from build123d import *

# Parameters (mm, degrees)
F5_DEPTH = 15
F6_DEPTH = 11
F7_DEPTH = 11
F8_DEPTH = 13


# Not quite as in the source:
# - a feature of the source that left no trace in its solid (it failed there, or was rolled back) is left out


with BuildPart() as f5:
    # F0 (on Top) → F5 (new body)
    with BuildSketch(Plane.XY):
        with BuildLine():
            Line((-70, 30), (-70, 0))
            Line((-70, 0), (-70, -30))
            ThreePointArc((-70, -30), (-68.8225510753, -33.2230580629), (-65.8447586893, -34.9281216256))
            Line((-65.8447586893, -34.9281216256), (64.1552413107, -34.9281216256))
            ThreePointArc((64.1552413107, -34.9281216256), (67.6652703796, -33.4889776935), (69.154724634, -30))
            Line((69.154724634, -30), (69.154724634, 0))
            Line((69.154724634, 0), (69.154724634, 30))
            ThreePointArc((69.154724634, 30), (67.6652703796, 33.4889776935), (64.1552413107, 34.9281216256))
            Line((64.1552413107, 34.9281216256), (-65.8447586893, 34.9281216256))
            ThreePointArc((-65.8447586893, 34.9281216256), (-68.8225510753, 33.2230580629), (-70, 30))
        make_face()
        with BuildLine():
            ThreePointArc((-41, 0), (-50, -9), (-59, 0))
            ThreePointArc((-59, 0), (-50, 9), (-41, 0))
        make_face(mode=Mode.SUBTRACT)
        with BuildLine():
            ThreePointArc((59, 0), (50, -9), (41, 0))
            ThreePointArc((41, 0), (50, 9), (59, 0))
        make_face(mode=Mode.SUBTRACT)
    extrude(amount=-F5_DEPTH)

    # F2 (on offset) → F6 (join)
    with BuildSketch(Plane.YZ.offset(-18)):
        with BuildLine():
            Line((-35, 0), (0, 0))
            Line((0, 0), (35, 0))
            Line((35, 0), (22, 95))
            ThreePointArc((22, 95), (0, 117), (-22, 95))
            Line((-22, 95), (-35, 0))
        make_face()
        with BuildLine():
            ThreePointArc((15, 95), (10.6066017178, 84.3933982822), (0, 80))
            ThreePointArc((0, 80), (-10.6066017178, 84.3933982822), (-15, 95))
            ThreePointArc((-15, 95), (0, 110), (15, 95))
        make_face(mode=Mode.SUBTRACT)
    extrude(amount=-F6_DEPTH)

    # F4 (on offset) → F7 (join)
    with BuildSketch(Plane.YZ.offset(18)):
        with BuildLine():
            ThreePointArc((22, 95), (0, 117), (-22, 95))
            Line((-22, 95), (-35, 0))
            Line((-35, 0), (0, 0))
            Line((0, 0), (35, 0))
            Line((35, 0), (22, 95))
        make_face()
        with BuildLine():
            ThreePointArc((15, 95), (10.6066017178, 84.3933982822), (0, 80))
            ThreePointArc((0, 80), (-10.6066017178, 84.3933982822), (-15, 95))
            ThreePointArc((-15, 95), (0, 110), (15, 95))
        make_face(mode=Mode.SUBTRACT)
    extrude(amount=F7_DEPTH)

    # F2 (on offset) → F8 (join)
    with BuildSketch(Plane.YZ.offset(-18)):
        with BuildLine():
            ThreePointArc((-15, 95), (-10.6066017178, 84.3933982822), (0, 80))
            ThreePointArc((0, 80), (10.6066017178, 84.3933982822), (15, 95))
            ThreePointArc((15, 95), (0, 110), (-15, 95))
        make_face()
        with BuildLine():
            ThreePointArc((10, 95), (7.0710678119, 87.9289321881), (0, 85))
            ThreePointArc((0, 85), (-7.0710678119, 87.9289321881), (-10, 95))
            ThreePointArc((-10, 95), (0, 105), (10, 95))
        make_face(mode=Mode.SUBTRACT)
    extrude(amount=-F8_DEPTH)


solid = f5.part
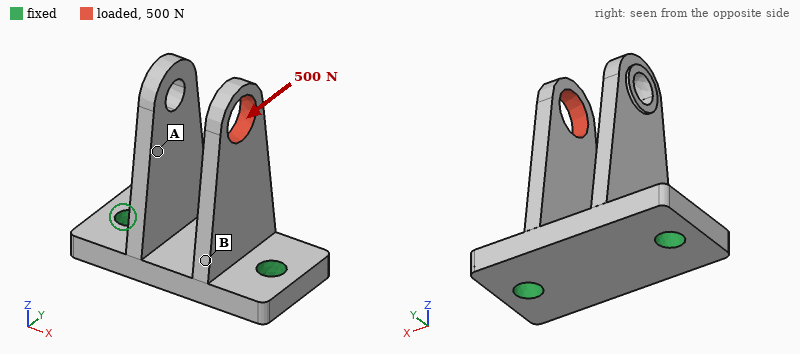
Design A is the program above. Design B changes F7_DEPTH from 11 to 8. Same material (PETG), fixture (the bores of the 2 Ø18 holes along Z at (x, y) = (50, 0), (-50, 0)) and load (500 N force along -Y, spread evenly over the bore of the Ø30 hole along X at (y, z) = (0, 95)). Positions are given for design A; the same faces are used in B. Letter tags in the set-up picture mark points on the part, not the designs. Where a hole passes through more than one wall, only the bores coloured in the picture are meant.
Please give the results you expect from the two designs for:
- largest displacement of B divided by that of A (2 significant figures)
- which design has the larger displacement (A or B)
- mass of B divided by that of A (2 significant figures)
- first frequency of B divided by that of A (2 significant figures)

1.2
B
0.94
0.88
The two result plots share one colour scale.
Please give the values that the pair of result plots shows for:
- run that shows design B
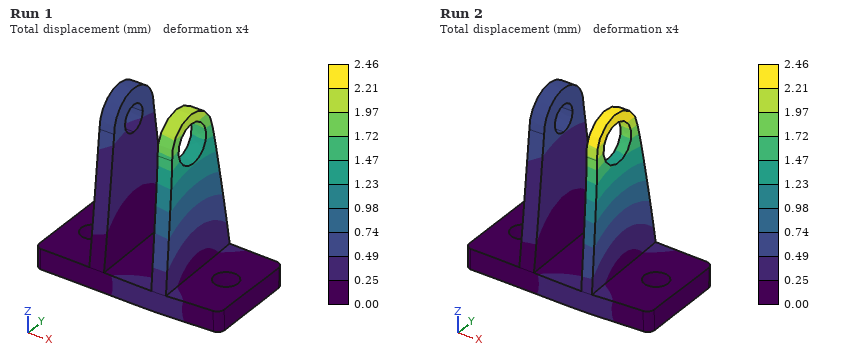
Run 2
